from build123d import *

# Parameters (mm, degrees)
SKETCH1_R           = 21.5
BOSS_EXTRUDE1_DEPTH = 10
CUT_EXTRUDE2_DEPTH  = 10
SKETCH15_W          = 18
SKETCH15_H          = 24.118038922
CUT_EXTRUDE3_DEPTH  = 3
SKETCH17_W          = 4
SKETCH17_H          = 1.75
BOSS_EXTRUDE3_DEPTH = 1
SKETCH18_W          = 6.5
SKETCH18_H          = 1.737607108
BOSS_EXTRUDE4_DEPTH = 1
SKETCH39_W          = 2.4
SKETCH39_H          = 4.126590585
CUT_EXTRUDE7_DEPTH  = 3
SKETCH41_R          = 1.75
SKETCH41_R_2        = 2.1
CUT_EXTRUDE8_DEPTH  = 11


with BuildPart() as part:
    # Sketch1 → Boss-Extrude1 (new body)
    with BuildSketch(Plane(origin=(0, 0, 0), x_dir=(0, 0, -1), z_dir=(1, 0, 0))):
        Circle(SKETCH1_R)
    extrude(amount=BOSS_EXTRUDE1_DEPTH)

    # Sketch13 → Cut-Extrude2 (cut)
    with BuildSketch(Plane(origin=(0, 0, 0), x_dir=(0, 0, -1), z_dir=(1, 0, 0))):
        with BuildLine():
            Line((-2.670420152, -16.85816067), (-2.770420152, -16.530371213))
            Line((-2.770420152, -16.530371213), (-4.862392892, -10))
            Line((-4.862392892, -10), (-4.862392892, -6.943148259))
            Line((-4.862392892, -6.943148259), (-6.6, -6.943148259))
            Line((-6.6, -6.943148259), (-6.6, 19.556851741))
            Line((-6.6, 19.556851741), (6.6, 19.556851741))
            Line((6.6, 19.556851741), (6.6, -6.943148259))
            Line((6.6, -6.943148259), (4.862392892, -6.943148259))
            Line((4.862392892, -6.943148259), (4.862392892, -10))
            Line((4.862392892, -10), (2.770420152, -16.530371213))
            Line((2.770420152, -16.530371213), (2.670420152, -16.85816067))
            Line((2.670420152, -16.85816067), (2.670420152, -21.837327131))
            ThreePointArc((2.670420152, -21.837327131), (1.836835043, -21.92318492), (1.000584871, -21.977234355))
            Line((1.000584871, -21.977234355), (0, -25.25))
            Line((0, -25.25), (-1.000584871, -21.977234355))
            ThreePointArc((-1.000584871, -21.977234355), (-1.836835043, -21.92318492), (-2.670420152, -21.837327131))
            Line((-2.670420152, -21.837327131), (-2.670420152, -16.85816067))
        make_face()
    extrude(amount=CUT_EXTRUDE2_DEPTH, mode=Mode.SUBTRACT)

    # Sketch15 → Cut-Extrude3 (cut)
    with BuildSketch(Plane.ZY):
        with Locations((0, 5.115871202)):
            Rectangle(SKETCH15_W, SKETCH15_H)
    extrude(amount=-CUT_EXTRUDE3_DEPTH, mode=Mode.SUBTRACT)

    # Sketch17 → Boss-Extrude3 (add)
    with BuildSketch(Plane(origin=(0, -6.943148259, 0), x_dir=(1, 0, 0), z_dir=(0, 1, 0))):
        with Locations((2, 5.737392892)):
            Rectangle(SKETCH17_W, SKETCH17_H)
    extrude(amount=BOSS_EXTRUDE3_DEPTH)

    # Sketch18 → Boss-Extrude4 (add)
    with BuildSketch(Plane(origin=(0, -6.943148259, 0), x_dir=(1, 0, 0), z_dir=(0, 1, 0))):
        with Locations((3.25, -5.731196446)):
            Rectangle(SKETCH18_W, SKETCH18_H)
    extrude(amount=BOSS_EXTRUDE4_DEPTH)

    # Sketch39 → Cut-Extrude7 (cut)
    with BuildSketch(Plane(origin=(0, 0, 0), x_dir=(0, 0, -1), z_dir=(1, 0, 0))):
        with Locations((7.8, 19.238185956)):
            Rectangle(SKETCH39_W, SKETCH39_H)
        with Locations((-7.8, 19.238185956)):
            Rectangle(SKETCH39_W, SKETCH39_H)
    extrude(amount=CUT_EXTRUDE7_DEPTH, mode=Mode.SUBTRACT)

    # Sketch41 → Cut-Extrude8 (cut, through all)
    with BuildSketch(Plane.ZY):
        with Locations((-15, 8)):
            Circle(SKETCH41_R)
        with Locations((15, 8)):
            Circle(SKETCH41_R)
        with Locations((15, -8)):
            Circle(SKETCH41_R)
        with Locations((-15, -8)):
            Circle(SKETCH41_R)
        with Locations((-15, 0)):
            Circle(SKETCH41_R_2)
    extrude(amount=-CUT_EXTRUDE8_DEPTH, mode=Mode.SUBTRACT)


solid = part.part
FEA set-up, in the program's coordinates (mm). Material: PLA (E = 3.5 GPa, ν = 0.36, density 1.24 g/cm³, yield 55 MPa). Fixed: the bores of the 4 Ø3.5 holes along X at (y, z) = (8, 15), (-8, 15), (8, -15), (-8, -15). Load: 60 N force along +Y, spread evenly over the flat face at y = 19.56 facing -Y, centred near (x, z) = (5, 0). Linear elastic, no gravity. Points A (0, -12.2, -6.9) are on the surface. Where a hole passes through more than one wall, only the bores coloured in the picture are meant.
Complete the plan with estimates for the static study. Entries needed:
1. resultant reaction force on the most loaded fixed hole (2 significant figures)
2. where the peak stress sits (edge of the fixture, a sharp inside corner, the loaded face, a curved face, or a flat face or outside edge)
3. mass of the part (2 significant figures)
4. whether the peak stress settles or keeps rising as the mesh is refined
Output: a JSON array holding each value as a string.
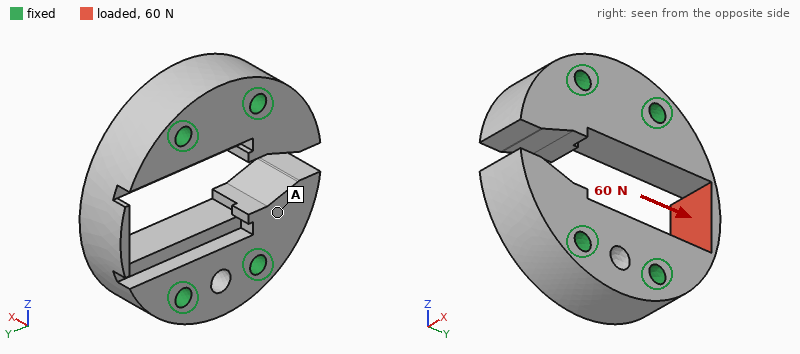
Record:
["41 N", "a sharp inside corner", "11 g", "keeps rising"]
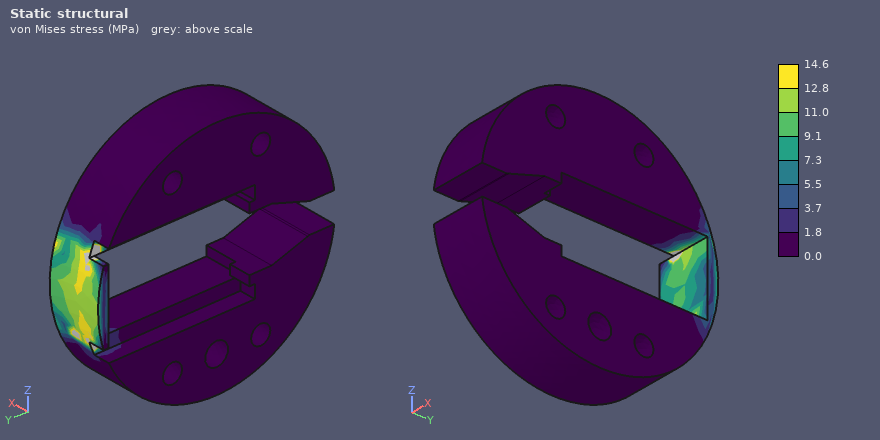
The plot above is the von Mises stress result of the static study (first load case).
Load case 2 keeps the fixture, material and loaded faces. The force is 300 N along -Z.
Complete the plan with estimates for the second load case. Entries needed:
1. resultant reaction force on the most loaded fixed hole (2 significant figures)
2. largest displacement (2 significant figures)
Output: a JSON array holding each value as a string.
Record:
["220 N", "0.22 mm"]
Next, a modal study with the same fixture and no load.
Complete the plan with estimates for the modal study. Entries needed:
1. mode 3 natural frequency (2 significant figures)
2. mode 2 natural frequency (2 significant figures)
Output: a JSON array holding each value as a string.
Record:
["9800 Hz", "9700 Hz"]
